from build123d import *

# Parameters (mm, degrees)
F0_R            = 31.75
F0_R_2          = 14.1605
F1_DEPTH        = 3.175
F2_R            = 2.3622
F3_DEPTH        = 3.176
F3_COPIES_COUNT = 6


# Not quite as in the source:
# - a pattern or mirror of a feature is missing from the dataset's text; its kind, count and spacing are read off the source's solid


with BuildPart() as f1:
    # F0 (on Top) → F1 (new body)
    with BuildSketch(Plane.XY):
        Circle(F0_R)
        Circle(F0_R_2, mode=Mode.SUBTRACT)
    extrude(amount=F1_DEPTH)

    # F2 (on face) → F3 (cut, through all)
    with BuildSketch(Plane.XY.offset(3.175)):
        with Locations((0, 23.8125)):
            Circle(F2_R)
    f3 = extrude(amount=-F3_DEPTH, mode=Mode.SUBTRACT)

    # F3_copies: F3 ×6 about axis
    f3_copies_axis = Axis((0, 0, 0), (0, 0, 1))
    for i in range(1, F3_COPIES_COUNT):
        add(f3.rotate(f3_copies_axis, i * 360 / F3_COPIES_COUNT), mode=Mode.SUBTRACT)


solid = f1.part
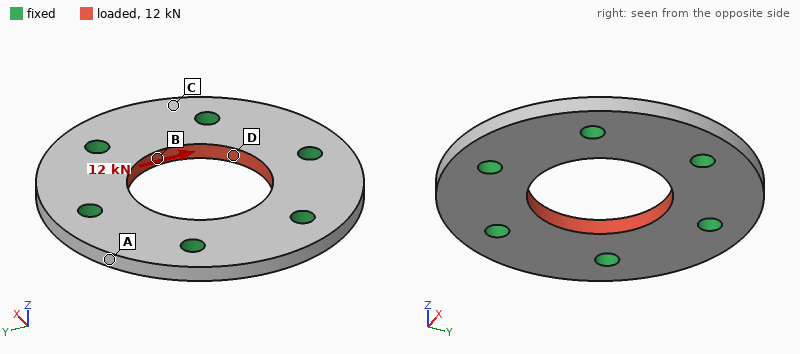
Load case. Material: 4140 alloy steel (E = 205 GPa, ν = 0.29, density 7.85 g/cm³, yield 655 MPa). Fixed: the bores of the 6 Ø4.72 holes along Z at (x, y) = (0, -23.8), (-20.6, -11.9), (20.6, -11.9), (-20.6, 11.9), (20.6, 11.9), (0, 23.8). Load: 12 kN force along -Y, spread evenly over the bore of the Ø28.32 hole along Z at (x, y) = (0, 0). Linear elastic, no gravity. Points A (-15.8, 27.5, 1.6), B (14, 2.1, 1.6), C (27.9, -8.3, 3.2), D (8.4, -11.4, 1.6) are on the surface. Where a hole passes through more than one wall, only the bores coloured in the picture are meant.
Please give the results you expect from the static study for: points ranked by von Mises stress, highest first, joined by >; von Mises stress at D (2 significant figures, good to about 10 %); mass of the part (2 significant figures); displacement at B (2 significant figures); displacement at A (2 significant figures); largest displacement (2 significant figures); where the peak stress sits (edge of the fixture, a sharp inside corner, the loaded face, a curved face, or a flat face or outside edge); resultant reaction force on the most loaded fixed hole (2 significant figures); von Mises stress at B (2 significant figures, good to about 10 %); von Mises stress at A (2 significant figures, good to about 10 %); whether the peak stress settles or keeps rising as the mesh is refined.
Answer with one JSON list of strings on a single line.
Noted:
["B > D > A > C", "56 MPa", "61 g", "2.9 µm", "1.6 µm", "3.6 µm", "edge of the fixture", "2.6 kN", "73 MPa", "22 MPa", "keeps rising"]
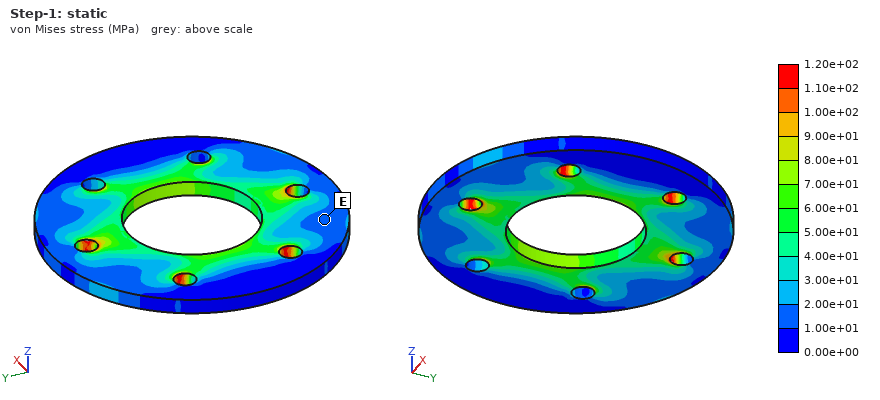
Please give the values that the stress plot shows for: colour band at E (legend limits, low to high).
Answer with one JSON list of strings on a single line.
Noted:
["1.00e+01 to 2.00e+01 MPa"]
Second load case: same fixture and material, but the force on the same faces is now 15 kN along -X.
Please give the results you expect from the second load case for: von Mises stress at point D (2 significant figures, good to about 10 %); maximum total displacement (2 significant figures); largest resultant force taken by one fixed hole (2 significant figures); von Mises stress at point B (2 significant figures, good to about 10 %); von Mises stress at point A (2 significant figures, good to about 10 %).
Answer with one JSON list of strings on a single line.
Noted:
["79 MPa", "4.5 µm", "2.9 kN", "52 MPa", "16 MPa"]
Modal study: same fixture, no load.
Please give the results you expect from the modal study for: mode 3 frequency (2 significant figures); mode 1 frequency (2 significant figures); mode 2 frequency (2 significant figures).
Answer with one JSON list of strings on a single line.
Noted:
["21 kHz", "21 kHz", "21 kHz"]
